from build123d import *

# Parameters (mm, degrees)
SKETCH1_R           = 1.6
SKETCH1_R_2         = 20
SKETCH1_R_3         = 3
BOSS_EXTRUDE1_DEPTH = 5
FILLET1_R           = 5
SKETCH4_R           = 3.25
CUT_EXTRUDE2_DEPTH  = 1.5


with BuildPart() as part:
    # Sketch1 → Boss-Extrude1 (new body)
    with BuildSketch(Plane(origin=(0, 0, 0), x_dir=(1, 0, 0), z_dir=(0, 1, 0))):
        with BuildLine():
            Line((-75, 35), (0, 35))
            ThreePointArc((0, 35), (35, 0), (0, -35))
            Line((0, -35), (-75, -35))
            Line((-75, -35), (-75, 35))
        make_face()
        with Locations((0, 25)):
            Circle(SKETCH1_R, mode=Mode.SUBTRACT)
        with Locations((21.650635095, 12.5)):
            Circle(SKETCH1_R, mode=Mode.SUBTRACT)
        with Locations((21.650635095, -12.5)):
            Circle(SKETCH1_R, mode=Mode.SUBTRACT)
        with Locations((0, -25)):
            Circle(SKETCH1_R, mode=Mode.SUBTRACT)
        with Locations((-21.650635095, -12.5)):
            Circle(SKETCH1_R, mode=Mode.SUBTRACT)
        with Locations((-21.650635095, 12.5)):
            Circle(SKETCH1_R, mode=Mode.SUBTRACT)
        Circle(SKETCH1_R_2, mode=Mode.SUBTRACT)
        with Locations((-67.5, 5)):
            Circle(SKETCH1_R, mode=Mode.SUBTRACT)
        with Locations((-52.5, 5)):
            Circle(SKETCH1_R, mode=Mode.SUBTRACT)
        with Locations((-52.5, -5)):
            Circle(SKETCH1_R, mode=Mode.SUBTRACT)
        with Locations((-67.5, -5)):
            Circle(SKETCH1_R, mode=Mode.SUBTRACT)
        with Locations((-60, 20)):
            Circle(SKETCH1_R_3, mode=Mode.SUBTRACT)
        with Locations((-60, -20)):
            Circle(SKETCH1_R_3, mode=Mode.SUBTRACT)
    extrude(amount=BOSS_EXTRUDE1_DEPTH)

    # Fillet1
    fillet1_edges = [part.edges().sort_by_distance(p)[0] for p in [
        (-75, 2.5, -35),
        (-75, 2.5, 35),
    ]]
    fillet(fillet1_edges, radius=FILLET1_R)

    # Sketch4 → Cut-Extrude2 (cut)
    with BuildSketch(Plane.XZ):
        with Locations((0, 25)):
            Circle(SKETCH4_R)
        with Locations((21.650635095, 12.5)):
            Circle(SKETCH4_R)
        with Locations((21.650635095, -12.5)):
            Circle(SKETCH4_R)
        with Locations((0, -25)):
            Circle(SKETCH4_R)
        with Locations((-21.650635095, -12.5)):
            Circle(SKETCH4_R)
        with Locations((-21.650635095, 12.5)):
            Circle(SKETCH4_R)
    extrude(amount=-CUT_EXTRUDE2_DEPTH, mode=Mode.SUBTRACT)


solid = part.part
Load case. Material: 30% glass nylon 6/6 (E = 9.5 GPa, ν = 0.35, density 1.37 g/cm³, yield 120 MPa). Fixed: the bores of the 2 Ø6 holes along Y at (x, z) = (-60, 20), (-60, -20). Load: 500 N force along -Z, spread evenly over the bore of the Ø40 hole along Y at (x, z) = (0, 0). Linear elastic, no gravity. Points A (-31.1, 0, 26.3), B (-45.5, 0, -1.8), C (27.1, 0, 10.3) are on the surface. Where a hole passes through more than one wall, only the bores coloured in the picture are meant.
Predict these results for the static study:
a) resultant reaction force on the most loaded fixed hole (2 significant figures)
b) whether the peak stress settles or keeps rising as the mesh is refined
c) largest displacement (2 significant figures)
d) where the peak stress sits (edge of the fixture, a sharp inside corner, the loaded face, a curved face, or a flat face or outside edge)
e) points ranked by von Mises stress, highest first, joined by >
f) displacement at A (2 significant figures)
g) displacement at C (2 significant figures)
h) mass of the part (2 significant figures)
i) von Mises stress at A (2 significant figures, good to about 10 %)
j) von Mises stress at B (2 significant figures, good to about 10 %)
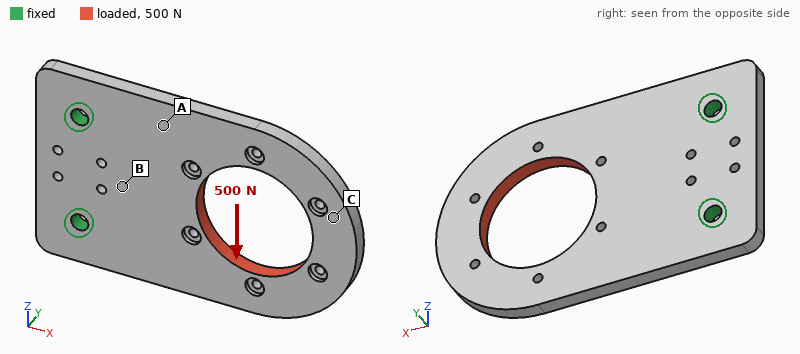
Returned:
730 N
keeps rising
0.18 mm
edge of the fixture
B > A > C
0.037 mm
0.17 mm
39 g
2.9 MPa
5.1 MPa
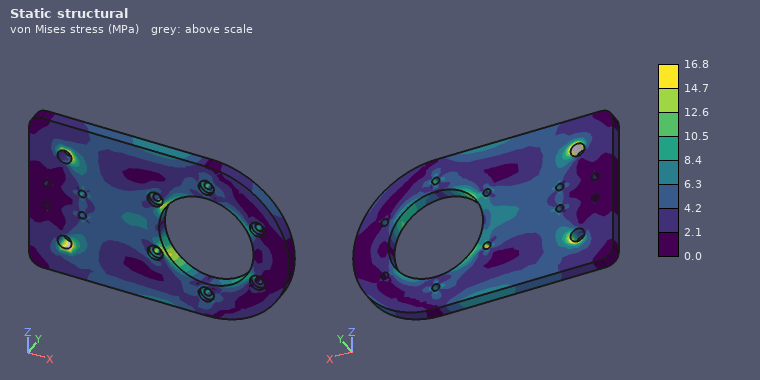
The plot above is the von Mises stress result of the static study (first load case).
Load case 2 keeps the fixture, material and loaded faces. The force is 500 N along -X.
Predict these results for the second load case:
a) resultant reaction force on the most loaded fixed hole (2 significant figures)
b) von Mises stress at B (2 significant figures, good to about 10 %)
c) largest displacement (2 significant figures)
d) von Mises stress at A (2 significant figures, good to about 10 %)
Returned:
250 N
0.57 MPa
33 µm
2.0 MPa
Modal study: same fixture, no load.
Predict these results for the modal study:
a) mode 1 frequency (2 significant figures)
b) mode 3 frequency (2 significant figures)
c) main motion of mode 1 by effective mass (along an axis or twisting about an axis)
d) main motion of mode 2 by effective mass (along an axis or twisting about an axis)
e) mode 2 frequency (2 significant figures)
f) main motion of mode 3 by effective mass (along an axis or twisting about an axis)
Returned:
300 Hz
1400 Hz
along Y
twisting about X
790 Hz
along Y
